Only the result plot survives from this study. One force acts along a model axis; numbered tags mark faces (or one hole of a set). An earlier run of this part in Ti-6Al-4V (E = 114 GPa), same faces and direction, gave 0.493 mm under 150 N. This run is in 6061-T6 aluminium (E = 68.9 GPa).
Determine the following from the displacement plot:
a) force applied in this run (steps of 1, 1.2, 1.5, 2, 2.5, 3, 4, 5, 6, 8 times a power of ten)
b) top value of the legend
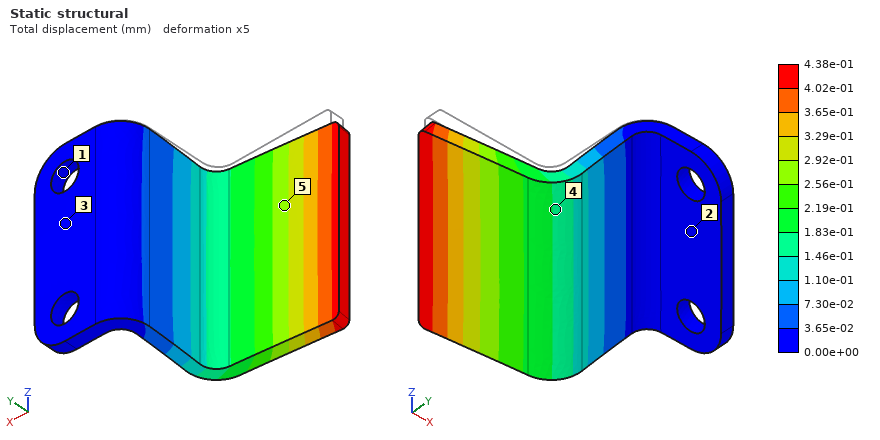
80 N
4.38e-01 mm
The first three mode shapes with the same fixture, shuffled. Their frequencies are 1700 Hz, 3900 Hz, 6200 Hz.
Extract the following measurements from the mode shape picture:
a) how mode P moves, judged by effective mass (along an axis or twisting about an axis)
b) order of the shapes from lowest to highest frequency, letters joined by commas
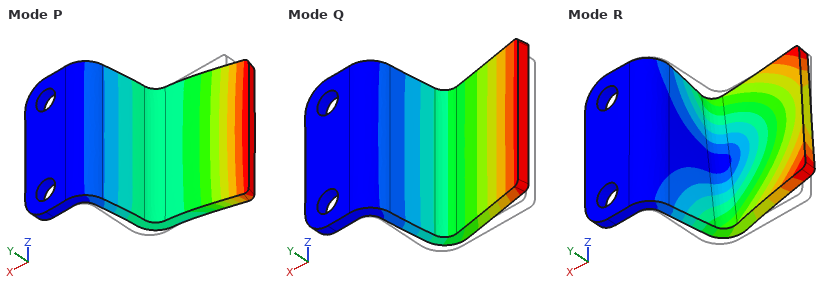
along X
Q, R, P
